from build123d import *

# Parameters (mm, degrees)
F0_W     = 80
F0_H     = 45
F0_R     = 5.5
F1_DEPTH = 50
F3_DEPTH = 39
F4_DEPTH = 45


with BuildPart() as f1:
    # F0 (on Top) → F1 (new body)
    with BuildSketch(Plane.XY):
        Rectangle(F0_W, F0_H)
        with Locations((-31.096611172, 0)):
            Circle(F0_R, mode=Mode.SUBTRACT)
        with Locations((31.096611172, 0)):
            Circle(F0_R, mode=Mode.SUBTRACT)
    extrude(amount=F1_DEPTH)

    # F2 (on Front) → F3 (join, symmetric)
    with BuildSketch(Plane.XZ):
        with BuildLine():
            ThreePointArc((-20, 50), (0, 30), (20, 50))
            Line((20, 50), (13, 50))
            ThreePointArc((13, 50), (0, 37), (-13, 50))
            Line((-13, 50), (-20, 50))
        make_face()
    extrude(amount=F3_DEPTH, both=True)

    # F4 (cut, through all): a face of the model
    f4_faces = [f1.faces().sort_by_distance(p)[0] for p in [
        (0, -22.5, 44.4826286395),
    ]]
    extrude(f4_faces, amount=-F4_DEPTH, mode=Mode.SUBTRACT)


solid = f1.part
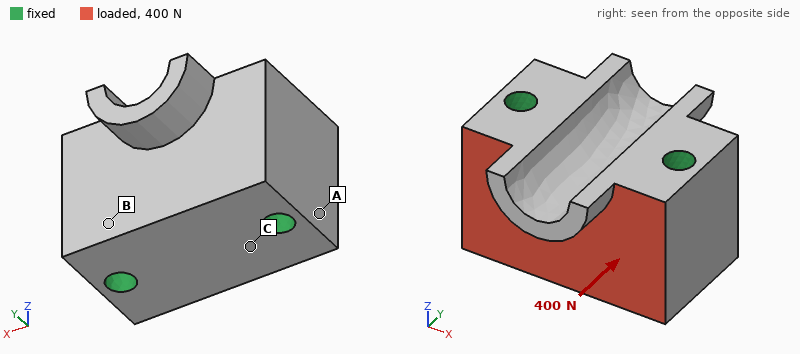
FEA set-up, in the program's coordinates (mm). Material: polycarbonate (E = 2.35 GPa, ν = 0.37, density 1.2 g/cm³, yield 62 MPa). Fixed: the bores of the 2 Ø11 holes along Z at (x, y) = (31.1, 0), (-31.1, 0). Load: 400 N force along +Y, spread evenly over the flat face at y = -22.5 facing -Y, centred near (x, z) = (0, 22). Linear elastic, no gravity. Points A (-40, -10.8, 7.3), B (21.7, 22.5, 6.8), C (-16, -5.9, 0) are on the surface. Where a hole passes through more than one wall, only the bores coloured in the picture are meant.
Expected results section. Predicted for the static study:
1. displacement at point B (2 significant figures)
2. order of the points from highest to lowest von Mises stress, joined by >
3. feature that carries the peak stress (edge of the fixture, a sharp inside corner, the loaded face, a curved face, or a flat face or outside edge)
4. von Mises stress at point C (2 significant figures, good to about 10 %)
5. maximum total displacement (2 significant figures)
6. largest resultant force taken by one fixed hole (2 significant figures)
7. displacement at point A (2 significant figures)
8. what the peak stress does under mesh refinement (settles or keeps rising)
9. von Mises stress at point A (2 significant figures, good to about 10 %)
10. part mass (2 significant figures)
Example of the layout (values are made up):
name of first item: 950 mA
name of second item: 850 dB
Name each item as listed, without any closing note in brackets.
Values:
displacement at point B: 1.0 µm
order of the points from highest to lowest von Mises stress, joined by >: C > A > B
feature that carries the peak stress: edge of the fixture
von Mises stress at point C: 0.13 MPa
maximum total displacement: 3.2 µm
largest resultant force taken by one fixed hole: 200 N
displacement at point A: 0.48 µm
what the peak stress does under mesh refinement: keeps rising
von Mises stress at point A: 0.075 MPa
part mass: 200 g
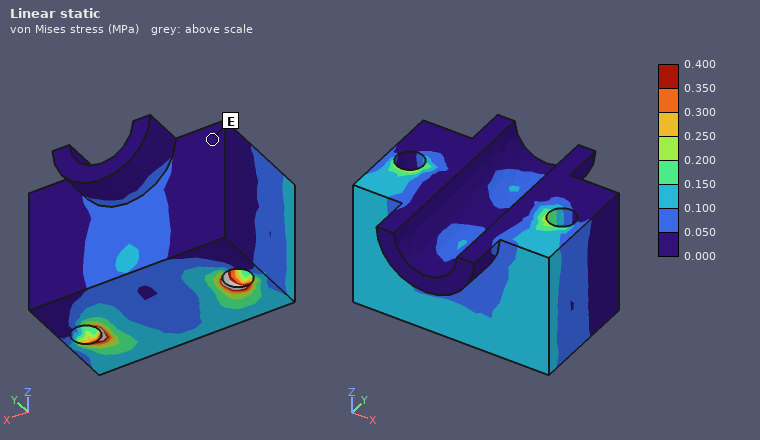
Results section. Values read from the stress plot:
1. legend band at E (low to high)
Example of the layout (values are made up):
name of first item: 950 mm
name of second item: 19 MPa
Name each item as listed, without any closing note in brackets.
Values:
legend band at E: 0.000 to 0.050 MPa
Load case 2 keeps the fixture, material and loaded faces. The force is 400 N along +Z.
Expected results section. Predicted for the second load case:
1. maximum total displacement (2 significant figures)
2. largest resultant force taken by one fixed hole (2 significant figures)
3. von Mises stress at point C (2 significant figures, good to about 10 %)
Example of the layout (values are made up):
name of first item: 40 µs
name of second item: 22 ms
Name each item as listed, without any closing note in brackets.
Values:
maximum total displacement: 7.9 µm
largest resultant force taken by one fixed hole: 200 N
von Mises stress at point C: 0.19 MPa
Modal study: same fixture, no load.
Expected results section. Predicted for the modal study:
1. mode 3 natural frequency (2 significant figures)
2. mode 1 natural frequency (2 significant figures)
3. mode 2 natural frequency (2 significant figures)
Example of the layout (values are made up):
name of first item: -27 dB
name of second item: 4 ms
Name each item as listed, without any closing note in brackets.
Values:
mode 3 natural frequency: 4700 Hz
mode 1 natural frequency: 4500 Hz
mode 2 natural frequency: 4600 Hz
